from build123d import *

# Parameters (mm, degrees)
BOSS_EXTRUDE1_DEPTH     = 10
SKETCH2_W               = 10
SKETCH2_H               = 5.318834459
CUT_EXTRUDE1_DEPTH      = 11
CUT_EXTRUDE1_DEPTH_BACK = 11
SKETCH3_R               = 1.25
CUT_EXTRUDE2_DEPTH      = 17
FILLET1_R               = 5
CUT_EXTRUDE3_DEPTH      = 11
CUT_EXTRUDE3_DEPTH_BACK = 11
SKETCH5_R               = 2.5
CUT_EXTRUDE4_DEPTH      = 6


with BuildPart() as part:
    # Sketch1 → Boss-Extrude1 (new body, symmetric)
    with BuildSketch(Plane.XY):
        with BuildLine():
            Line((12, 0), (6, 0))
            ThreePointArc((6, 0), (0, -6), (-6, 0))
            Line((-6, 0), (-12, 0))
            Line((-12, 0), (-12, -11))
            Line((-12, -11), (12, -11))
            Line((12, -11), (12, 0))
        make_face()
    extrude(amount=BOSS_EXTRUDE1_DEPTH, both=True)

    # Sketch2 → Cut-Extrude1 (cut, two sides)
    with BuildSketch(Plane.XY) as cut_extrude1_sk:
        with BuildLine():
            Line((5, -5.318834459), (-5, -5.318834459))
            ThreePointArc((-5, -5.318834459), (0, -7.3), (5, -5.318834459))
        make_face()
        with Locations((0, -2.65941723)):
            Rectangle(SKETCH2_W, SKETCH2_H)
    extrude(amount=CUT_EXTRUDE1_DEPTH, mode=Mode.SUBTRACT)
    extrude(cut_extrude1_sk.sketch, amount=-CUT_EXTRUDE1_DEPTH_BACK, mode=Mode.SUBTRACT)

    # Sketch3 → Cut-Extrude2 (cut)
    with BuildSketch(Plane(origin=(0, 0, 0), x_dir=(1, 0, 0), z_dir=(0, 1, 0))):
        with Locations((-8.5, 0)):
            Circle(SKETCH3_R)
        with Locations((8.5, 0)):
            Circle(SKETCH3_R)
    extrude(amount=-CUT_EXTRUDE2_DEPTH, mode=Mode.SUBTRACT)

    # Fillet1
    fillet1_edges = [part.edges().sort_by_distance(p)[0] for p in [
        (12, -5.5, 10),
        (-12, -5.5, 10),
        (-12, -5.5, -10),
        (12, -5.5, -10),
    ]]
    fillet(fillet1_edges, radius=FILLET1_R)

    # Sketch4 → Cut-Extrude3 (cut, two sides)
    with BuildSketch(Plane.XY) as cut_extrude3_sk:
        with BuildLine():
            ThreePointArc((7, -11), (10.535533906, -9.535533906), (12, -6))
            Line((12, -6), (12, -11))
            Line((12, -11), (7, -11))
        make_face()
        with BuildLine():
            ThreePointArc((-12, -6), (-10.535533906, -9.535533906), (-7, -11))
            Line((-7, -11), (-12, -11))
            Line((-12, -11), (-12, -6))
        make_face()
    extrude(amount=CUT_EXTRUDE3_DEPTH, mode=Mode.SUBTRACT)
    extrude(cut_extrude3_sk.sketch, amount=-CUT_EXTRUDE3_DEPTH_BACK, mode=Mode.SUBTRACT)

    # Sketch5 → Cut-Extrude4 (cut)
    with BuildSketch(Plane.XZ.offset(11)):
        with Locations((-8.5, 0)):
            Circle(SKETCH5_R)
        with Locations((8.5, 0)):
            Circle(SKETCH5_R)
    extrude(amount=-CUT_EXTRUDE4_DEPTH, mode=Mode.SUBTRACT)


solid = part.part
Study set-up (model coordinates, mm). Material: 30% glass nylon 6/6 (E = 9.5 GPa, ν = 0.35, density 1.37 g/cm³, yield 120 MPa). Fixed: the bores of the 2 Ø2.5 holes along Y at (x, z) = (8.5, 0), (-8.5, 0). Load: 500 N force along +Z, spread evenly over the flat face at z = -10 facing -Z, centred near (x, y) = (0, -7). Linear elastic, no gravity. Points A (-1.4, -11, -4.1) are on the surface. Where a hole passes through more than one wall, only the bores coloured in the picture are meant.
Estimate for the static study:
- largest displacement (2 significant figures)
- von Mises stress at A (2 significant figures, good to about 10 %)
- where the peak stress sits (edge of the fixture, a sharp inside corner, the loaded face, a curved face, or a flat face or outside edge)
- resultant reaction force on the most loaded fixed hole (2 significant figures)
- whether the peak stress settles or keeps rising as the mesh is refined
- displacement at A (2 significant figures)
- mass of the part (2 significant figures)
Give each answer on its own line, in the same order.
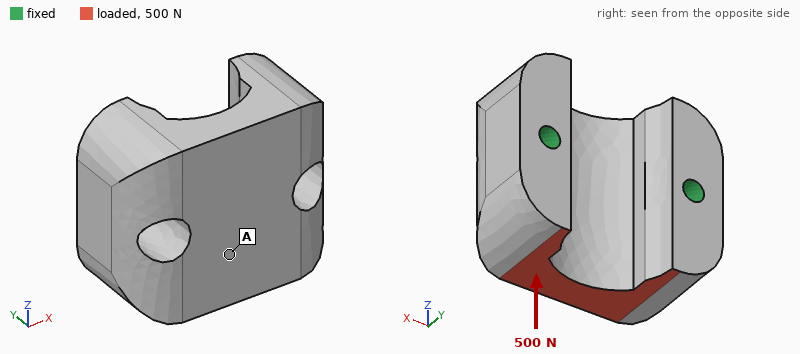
50 µm
7.5 MPa
edge of the fixture
250 N
keeps rising
35 µm
4.4 g
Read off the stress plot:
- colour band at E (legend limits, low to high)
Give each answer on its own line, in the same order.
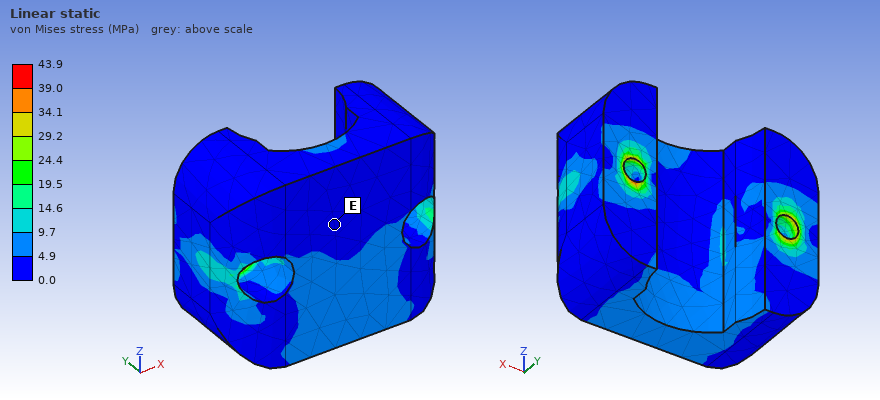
0.0 to 4.9 MPa
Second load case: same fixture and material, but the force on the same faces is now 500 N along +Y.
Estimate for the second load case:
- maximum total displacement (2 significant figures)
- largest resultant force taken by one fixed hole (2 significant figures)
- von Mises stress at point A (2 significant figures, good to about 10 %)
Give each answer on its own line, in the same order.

0.12 mm
280 N
15 MPa
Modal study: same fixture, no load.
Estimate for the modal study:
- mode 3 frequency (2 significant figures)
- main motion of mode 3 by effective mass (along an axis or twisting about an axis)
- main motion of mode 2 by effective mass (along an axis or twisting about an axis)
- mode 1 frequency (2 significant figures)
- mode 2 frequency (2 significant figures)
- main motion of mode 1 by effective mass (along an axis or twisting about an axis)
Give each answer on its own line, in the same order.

18 kHz
along X
twisting about Y
9700 Hz
15 kHz
along Z
